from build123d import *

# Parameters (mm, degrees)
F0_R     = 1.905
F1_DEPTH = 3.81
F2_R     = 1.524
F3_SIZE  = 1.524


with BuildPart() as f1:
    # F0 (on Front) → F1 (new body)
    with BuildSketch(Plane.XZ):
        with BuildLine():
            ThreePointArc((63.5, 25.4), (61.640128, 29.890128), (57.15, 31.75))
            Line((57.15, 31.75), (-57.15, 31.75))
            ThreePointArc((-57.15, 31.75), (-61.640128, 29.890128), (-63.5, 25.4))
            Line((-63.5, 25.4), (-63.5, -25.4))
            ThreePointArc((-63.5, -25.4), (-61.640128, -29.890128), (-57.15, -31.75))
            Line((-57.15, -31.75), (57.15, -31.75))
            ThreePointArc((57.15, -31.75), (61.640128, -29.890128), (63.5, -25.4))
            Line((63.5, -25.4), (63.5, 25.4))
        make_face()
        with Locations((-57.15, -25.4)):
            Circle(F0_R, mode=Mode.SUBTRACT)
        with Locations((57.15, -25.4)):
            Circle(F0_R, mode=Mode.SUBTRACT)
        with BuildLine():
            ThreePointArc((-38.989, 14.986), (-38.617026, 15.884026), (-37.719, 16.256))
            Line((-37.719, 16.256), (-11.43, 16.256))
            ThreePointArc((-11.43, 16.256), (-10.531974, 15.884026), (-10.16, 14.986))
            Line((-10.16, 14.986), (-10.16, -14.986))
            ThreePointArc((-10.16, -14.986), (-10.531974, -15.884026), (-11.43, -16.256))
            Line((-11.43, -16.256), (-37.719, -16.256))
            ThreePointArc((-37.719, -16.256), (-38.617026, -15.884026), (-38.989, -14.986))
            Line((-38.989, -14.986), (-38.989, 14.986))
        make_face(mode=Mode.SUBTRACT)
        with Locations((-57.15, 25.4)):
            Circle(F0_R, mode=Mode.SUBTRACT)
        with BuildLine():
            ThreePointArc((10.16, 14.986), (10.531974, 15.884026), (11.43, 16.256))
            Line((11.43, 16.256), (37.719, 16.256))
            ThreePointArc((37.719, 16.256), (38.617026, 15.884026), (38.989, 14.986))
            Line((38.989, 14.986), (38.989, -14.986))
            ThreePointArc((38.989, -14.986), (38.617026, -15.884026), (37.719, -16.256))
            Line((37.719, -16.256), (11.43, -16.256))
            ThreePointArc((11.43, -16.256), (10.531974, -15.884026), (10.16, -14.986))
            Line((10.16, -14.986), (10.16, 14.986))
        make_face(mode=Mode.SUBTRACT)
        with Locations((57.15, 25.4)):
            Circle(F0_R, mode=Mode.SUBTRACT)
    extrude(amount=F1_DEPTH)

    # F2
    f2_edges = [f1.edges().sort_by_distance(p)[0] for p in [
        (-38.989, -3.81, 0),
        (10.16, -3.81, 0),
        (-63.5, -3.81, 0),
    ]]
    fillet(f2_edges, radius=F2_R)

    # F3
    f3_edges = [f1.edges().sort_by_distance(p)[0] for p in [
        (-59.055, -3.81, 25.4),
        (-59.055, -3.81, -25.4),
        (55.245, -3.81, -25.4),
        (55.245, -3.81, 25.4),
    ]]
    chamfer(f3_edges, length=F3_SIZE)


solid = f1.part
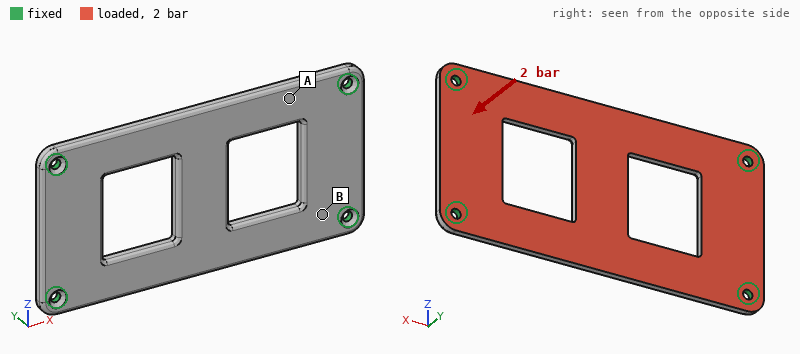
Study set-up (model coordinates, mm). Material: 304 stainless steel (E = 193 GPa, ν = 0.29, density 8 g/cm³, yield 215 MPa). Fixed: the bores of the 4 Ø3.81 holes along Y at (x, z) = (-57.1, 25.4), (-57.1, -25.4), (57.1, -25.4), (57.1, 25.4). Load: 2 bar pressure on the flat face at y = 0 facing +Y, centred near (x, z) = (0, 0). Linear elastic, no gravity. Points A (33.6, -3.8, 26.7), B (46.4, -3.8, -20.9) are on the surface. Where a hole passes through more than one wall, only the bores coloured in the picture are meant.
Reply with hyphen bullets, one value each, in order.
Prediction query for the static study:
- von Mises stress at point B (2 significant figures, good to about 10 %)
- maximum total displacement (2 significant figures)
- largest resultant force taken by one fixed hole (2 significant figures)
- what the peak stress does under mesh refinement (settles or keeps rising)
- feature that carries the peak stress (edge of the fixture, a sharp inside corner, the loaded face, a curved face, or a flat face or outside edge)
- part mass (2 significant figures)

- 34 MPa
- 0.14 mm
- 350 N
- keeps rising
- edge of the fixture
- 180 g
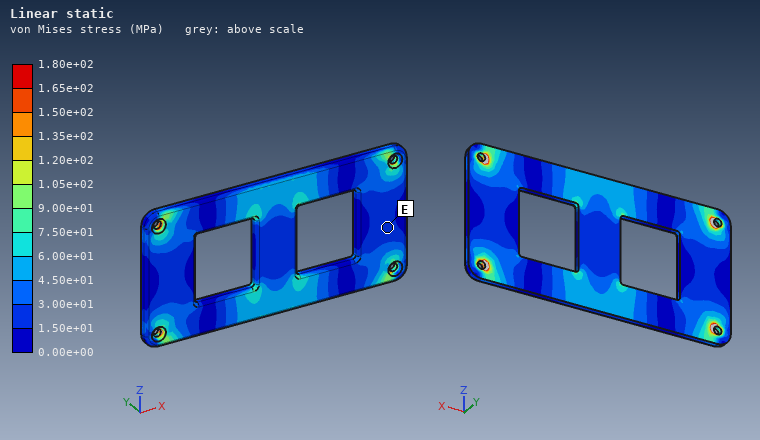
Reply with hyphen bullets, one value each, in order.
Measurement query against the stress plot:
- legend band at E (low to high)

- 1.50e+01 to 3.00e+01 MPa
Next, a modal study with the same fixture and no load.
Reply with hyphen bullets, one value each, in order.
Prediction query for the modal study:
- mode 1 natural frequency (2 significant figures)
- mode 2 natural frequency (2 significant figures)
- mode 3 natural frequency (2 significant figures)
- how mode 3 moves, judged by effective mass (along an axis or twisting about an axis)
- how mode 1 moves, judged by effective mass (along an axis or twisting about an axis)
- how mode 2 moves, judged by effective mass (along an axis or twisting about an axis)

- 1200 Hz
- 1900 Hz
- 3500 Hz
- twisting about Z
- along Y
- twisting about X
